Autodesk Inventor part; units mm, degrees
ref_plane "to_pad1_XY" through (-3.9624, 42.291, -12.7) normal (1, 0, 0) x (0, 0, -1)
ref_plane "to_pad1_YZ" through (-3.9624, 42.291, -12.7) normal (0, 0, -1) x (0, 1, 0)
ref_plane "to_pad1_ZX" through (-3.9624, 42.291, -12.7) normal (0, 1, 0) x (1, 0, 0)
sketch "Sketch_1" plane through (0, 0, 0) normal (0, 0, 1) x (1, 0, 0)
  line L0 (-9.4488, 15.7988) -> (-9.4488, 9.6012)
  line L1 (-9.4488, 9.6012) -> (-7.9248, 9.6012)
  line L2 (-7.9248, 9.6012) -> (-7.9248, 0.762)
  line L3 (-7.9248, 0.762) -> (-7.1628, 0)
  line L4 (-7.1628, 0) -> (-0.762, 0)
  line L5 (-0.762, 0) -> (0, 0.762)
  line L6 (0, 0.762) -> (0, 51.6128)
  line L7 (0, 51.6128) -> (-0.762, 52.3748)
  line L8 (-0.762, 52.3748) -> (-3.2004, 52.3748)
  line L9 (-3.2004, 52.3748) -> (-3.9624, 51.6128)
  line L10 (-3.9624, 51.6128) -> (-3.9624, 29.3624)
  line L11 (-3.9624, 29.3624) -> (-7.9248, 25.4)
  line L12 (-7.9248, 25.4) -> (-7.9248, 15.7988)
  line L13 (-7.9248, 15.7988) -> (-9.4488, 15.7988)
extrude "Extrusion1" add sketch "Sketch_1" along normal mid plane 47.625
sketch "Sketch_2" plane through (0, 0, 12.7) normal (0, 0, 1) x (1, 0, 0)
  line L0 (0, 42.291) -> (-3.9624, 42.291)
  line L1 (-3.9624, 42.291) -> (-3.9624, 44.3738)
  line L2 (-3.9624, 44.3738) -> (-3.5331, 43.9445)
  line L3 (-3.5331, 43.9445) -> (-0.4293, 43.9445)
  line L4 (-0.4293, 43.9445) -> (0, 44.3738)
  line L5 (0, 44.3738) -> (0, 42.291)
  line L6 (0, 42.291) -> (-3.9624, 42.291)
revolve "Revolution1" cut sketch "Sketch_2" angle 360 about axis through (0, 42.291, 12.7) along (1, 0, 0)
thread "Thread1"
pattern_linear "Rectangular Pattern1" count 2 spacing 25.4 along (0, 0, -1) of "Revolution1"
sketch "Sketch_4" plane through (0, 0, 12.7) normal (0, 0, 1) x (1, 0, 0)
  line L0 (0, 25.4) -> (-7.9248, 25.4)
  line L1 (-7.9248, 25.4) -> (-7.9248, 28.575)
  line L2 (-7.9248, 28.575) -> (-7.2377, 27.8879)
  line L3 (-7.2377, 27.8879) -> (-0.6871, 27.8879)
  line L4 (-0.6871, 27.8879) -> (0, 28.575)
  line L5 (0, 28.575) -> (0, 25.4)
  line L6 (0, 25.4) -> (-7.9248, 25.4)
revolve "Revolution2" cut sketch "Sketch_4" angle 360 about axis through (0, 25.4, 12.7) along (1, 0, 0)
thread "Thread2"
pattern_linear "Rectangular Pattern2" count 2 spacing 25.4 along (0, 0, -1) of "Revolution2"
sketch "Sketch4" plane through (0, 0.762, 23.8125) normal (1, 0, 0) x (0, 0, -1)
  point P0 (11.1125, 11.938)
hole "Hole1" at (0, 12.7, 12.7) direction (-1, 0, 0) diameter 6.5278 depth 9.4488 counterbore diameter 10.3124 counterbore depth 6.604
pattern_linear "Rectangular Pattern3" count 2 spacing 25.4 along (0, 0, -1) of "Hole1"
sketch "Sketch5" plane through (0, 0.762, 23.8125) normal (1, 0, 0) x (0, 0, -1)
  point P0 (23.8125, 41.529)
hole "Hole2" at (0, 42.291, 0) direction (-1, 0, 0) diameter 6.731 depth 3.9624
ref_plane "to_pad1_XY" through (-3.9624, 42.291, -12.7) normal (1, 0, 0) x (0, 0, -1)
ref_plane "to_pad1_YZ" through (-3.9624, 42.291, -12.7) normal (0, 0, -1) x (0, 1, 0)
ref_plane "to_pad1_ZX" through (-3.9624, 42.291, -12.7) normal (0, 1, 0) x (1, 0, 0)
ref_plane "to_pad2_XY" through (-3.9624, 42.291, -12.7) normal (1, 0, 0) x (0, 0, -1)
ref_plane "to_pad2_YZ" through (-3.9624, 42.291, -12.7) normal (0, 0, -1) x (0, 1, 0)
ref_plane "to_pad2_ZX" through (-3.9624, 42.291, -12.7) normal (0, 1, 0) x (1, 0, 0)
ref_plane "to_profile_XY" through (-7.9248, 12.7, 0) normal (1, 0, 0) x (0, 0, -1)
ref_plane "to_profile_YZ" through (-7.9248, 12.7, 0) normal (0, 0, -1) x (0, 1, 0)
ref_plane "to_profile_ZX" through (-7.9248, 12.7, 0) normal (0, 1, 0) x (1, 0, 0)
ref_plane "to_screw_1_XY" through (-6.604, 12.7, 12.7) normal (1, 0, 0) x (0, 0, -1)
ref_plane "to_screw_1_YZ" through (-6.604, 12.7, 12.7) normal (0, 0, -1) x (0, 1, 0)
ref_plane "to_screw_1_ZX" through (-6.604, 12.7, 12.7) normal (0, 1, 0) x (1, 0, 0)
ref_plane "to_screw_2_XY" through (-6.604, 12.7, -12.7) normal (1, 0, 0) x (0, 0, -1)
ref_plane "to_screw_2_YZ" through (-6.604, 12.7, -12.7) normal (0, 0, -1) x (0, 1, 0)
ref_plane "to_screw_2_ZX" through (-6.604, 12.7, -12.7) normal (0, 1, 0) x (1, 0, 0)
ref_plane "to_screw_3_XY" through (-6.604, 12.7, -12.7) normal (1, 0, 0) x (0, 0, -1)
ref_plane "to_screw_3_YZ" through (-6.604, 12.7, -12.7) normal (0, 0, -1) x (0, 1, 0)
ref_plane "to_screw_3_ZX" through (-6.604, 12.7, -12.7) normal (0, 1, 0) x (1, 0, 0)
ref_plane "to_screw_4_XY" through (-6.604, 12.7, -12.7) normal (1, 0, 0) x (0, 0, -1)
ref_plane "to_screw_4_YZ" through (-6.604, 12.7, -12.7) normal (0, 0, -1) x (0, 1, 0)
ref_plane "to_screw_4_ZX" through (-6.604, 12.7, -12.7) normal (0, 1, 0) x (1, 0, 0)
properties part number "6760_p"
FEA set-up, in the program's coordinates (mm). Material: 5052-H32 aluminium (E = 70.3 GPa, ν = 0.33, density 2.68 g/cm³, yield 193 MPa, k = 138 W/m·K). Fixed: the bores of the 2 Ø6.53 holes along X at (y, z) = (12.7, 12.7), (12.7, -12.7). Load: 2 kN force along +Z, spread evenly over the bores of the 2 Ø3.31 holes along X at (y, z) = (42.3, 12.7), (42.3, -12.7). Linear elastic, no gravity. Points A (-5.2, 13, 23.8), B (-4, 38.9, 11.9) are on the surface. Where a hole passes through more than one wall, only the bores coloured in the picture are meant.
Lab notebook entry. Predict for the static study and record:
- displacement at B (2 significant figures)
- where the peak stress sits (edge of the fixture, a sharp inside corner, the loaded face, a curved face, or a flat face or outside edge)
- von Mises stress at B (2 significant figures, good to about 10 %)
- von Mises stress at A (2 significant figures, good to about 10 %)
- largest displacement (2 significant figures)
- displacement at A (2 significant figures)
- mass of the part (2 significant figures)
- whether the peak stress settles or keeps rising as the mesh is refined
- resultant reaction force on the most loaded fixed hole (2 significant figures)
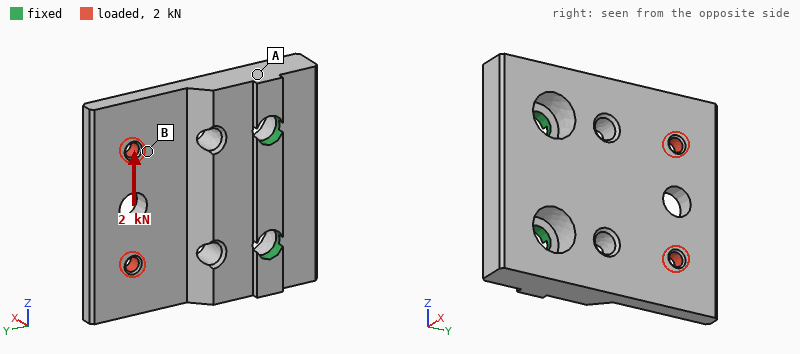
33 µm
edge of the fixture
34 MPa
17 MPa
55 µm
13 µm
37 g
keeps rising
2.3 kN
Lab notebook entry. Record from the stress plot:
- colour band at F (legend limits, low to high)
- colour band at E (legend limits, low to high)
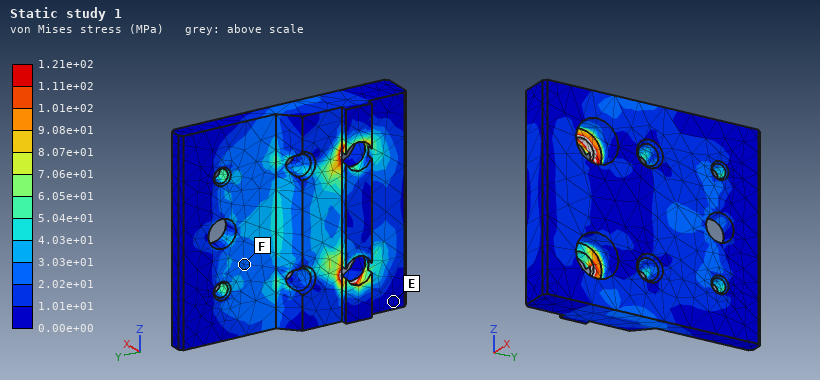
2.02e+01 to 3.03e+01 MPa
0.00e+00 to 1.01e+01 MPa
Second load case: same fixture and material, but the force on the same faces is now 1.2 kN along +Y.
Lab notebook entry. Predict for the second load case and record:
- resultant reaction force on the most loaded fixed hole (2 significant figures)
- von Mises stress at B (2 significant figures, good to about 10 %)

600 N
11 MPa
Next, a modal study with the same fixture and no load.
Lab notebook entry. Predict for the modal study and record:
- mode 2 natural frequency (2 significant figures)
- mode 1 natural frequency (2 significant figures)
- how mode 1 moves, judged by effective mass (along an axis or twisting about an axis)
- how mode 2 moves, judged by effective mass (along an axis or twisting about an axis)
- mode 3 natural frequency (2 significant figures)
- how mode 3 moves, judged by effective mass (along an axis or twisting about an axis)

5600 Hz
2500 Hz
along X
twisting about Y
9500 Hz
along Y
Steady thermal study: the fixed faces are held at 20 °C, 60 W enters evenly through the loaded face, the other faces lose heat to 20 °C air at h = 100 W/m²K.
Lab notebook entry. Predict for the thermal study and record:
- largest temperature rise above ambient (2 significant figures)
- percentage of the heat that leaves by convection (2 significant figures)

66 K
28 %
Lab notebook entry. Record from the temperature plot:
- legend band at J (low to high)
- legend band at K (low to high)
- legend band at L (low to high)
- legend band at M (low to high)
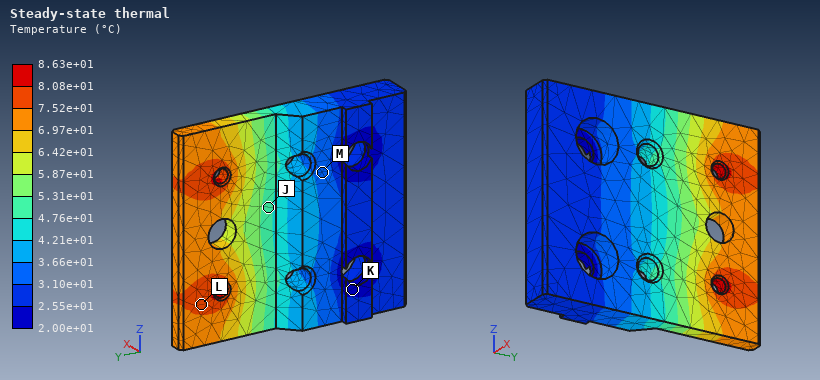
4.76e+01 to 5.31e+01 °C
2.00e+01 to 2.55e+01 °C
7.52e+01 to 8.08e+01 °C
3.10e+01 to 3.66e+01 °C
